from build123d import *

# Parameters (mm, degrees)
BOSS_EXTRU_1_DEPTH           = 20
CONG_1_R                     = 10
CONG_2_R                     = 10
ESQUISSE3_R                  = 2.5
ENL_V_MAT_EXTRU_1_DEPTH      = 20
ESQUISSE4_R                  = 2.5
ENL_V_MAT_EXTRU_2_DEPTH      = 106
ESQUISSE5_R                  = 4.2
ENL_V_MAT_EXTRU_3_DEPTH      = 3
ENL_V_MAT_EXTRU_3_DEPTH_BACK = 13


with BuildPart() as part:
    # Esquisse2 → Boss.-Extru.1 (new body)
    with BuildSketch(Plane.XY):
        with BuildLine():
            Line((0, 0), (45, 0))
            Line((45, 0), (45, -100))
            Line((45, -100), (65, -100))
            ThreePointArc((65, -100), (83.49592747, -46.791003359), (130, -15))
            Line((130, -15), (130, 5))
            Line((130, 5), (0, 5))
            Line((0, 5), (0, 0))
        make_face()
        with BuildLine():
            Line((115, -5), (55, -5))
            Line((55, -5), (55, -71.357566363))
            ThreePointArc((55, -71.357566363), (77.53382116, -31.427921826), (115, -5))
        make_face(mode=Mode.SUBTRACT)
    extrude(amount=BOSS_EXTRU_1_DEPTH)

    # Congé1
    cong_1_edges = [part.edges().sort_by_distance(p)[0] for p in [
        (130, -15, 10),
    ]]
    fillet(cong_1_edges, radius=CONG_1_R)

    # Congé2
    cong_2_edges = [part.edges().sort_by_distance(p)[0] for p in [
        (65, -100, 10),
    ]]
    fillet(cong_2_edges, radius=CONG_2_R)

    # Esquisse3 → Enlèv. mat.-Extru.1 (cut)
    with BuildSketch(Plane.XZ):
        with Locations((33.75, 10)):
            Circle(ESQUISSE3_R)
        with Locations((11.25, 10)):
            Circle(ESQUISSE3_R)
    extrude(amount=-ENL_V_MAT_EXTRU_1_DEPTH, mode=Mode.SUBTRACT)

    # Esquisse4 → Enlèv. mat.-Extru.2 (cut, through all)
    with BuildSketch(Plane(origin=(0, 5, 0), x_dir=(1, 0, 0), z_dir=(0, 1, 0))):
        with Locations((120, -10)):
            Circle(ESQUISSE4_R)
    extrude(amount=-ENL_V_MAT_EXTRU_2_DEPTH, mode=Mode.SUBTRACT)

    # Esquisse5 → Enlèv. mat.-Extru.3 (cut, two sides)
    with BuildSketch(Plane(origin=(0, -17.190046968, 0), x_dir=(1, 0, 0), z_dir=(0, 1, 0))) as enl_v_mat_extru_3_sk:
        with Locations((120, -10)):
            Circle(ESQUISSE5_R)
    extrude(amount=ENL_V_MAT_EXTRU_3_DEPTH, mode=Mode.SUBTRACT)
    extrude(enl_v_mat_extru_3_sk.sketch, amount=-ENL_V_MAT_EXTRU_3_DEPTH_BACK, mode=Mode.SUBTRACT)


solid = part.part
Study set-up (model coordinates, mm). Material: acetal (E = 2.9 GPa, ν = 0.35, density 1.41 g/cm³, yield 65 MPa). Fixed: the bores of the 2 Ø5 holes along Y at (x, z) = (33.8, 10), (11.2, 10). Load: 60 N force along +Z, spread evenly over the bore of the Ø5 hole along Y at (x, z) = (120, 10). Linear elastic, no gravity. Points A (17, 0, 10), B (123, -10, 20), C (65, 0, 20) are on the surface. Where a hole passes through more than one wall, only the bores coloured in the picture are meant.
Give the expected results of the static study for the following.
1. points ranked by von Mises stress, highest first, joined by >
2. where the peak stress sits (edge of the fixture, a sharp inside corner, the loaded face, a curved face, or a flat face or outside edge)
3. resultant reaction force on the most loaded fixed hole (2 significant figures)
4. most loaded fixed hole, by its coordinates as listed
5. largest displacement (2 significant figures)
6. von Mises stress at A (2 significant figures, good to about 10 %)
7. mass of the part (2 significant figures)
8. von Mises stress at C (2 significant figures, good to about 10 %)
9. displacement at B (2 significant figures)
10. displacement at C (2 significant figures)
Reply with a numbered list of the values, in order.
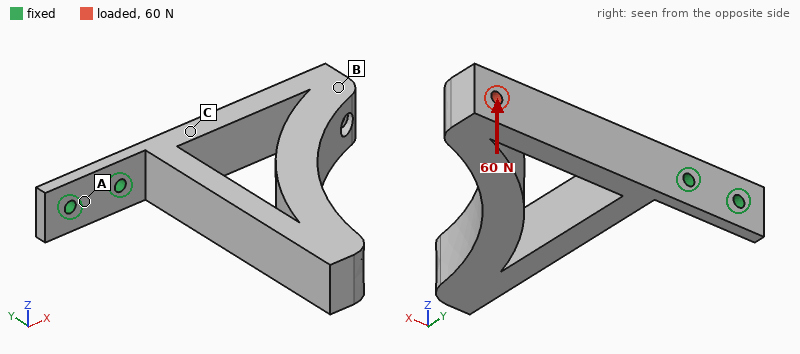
1. C > A > B
2. edge of the fixture
3. 200 N
4. (33.8, 10)
5. 1.5 mm
6. 2.9 MPa
7. 100 g
8. 4.6 MPa
9. 1.4 mm
10. 0.38 mm
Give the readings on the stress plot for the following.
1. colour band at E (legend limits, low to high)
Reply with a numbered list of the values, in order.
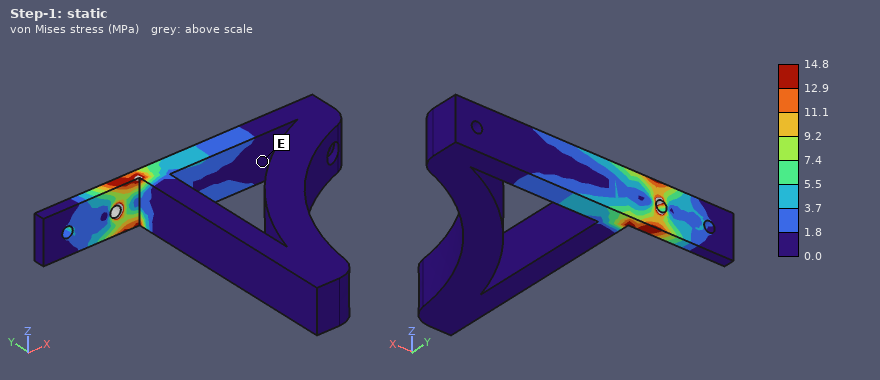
1. 0.0 to 1.8 MPa
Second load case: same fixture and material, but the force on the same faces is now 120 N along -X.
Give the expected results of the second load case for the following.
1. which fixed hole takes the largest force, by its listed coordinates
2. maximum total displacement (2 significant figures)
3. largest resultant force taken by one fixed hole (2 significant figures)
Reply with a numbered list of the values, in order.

1. (33.8, 10)
2. 1.9 mm
3. 110 N
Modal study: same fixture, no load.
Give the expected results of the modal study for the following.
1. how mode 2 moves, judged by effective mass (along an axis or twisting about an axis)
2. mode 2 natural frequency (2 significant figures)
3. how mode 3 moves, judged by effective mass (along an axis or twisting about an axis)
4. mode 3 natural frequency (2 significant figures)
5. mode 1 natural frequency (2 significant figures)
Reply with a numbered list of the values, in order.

1. along Z
2. 91 Hz
3. along Z
4. 230 Hz
5. 53 Hz
